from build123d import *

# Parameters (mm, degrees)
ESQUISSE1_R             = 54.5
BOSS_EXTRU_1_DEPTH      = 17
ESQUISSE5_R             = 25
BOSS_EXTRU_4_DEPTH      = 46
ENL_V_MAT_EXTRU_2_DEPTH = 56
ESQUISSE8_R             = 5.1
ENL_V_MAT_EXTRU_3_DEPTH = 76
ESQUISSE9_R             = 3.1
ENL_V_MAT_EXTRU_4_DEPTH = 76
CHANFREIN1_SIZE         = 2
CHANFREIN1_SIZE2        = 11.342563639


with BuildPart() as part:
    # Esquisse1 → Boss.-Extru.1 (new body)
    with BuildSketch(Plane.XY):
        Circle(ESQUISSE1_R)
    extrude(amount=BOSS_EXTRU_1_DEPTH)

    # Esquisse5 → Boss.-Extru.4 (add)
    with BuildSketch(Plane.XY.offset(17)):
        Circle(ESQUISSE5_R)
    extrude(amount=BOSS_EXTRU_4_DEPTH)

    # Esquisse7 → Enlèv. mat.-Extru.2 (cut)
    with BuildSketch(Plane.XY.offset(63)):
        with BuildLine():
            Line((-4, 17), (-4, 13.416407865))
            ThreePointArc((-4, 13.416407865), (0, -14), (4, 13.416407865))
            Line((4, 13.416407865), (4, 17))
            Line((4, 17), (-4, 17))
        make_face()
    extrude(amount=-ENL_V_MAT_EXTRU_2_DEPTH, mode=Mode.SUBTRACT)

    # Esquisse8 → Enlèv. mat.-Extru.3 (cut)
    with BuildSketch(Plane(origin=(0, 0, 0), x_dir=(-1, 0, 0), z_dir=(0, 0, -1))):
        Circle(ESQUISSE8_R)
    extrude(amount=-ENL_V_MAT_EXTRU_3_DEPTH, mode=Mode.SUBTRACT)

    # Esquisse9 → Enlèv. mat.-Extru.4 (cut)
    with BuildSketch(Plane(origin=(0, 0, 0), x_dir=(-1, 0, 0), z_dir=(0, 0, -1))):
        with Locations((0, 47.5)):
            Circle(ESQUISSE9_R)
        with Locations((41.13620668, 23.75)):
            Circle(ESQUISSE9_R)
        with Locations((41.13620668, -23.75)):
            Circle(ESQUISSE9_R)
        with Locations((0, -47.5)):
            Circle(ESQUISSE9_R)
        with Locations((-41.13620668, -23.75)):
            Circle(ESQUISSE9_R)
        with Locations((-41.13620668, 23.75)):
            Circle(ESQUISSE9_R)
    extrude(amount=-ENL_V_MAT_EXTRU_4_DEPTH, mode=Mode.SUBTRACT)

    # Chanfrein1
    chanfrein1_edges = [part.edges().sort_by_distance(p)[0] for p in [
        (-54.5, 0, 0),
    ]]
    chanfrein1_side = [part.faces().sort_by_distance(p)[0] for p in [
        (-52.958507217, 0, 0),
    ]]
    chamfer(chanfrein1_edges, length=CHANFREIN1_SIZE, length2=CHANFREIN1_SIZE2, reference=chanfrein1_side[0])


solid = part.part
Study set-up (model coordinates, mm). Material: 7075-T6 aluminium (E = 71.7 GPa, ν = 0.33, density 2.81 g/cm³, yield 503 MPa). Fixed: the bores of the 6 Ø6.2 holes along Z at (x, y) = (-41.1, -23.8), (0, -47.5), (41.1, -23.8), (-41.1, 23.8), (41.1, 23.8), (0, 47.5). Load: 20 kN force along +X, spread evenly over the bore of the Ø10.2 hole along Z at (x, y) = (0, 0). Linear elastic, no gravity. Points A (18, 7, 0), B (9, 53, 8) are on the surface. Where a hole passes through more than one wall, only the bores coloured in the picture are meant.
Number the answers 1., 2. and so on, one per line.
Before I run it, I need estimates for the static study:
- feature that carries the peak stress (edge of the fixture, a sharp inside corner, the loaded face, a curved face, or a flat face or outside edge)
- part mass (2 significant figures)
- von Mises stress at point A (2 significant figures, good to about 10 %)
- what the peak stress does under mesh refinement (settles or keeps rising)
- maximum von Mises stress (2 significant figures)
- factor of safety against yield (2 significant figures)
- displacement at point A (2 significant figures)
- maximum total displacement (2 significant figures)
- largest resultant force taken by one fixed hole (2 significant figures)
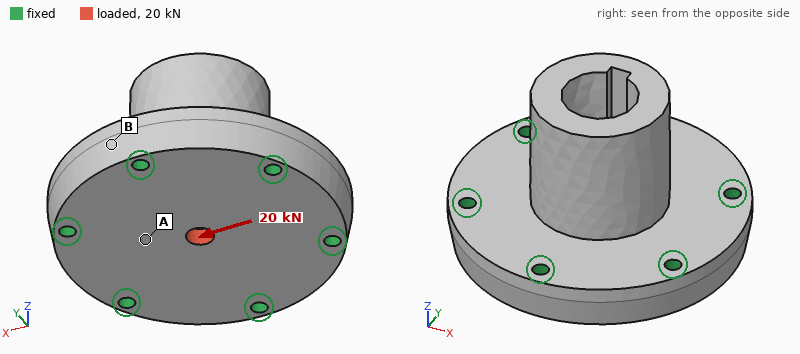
1. the loaded face
2. 580 g
3. 35 MPa
4. settles
5. 160 MPa
6. 3.2
7. 8.6 µm
8. 21 µm
9. 4.6 kN
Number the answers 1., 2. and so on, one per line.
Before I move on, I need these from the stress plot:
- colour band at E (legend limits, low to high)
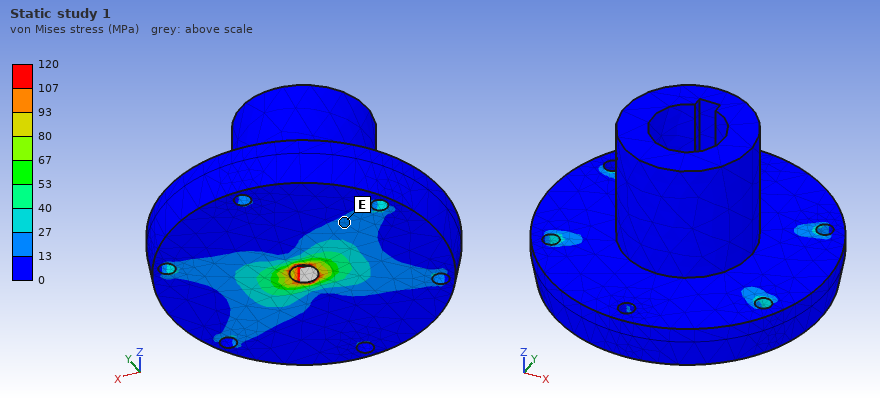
1. 13 to 27 MPa
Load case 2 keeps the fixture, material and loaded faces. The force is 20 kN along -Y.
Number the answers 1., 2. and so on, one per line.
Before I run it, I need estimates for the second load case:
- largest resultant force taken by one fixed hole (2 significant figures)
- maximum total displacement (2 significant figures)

1. 5.2 kN
2. 21 µm
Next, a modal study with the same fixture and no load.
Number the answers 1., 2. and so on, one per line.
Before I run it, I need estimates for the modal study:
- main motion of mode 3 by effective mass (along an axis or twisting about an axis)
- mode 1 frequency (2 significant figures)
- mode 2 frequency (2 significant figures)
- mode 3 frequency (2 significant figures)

1. along Z
2. 7000 Hz
3. 7000 Hz
4. 9200 Hz
